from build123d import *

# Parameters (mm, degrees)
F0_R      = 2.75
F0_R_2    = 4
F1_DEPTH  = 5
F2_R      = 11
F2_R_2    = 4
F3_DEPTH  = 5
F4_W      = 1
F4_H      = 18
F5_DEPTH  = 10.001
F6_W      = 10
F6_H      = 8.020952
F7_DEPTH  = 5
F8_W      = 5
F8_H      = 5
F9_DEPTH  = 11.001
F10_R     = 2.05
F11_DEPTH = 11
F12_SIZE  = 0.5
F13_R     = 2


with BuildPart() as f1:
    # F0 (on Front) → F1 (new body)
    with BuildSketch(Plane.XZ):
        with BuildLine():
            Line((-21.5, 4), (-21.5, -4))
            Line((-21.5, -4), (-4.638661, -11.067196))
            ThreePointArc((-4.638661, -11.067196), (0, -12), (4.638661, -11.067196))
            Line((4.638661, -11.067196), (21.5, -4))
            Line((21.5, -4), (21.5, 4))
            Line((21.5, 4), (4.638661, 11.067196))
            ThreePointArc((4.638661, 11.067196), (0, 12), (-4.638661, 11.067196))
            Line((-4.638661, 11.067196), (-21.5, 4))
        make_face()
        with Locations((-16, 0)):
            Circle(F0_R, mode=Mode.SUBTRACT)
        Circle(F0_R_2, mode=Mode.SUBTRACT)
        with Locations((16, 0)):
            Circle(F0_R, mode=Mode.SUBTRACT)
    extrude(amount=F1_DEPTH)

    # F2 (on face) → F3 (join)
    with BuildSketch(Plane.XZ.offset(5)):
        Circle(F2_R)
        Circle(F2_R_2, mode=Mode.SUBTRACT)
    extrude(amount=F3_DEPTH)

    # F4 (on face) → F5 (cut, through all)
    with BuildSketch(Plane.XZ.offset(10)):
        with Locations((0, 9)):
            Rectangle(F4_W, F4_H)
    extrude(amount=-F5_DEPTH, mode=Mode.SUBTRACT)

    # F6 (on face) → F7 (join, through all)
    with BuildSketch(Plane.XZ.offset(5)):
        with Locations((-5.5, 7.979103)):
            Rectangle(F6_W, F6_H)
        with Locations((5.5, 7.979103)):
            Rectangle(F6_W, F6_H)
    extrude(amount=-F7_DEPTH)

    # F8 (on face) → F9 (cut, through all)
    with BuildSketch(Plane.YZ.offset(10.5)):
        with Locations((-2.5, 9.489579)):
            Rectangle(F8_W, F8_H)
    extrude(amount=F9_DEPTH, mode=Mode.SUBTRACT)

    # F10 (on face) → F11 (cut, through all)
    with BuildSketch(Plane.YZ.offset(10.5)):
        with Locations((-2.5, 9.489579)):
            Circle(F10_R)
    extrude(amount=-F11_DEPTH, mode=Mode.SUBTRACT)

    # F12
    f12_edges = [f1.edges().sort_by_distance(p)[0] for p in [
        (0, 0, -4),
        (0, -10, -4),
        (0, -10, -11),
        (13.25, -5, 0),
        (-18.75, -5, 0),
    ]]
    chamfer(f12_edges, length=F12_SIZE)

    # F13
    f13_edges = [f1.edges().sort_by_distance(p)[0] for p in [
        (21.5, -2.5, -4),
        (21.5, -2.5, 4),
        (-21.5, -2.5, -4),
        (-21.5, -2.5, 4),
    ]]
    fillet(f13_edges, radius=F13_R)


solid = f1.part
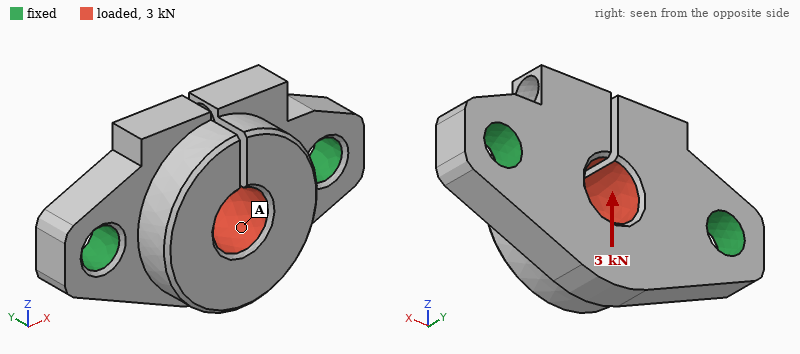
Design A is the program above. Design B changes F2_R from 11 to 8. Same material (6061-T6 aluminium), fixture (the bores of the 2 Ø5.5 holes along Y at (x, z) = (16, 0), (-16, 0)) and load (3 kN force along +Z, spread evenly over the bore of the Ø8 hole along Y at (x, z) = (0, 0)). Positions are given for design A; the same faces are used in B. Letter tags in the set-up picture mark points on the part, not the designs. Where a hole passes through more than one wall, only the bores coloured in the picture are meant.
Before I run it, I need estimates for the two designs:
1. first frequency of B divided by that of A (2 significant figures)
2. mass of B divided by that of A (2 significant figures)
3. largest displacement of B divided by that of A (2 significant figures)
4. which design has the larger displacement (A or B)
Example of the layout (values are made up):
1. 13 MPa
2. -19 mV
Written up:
1. 1.0
2. 0.81
3. 1.2
4. B
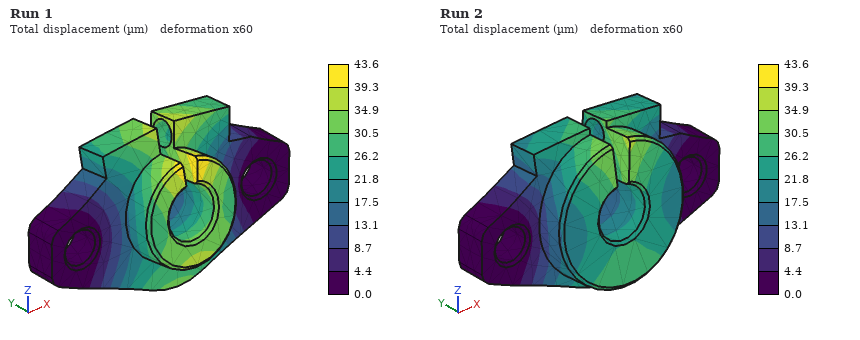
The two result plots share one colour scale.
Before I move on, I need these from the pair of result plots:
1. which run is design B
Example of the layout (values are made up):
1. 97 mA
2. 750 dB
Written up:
1. Run 1
